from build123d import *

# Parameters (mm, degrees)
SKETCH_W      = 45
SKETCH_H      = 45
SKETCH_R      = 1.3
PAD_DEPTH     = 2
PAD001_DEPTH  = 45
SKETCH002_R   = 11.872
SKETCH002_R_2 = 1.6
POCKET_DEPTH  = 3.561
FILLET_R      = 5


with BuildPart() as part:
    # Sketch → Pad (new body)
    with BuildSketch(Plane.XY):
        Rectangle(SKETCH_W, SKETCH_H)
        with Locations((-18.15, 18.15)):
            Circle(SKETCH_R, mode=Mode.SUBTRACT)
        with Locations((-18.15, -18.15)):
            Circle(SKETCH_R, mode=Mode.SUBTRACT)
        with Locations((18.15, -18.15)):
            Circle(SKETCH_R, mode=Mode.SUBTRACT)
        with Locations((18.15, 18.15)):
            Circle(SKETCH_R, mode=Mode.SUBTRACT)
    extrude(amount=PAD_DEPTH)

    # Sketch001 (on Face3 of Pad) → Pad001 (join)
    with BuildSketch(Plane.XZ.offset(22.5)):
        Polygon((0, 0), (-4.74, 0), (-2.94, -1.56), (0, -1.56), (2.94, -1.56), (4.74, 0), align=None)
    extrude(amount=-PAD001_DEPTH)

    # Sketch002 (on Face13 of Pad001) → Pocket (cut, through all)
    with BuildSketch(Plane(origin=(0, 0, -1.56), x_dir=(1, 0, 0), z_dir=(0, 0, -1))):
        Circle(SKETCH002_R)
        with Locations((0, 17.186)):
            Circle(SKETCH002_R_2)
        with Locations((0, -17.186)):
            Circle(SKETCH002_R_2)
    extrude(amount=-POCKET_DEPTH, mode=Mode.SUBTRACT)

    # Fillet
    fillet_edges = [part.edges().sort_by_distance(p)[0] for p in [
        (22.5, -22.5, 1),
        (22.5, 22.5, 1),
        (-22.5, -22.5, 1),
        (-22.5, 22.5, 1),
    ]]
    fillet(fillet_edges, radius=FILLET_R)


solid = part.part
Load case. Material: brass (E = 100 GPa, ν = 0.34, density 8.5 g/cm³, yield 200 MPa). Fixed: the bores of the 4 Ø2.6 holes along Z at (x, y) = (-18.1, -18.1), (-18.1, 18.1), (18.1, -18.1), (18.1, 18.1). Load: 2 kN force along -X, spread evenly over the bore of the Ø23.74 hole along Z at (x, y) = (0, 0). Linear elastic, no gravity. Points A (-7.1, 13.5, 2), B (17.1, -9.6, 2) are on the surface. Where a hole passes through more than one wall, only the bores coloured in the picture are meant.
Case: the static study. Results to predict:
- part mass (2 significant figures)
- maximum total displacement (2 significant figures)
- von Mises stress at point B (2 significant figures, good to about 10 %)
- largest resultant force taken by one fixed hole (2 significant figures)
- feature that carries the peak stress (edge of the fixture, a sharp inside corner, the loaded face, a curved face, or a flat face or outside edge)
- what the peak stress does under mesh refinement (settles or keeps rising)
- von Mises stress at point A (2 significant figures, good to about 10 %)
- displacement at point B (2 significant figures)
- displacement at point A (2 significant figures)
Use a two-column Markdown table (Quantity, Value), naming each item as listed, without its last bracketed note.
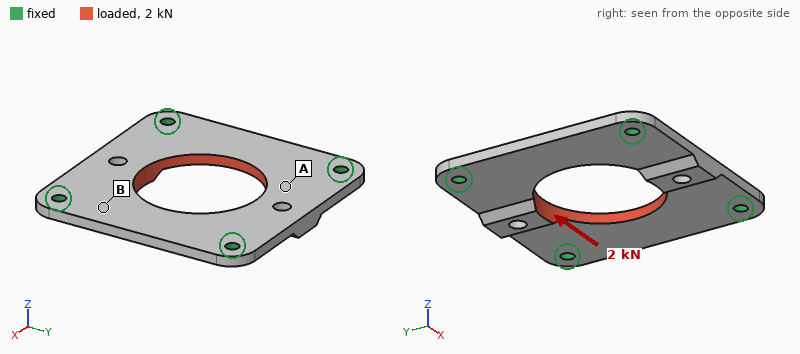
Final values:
| Quantity | Value |
|---|---|
| part mass | 28 g |
| maximum total displacement | 7.2 µm |
| von Mises stress at point B | 15 MPa |
| largest resultant force taken by one fixed hole | 530 N |
| feature that carries the peak stress | edge of the fixture |
| what the peak stress does under mesh refinement | keeps rising |
| von Mises stress at point A | 20 MPa |
| displacement at point B | 4.3 µm |
| displacement at point A | 3.5 µm |
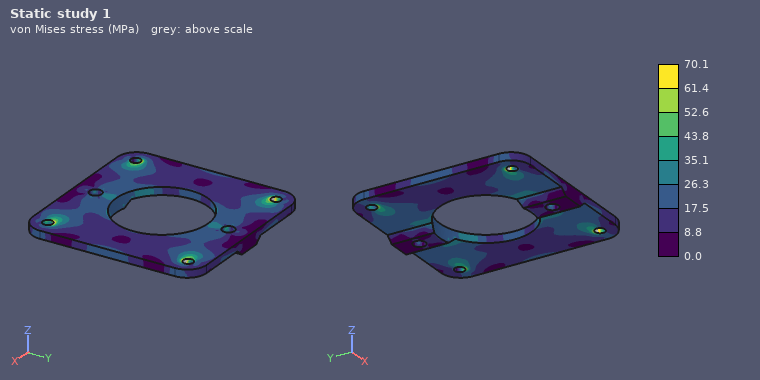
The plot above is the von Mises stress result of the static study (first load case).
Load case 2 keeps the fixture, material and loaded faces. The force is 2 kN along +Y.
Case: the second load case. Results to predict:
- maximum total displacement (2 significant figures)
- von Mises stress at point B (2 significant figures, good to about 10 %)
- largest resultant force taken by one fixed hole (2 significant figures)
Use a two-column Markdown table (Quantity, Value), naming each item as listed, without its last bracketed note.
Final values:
| Quantity | Value |
|---|---|
| maximum total displacement | 13 µm |
| von Mises stress at point B | 20 MPa |
| largest resultant force taken by one fixed hole | 530 N |
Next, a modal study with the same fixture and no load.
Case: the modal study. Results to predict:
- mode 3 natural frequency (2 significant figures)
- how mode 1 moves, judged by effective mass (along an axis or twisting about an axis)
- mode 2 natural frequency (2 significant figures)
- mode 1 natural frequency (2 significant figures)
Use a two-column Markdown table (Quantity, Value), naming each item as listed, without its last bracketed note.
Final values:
| Quantity | Value |
|---|---|
| mode 3 natural frequency | 6000 Hz |
| how mode 1 moves, judged by effective mass | along Z |
| mode 2 natural frequency | 5900 Hz |
| mode 1 natural frequency | 4800 Hz |
